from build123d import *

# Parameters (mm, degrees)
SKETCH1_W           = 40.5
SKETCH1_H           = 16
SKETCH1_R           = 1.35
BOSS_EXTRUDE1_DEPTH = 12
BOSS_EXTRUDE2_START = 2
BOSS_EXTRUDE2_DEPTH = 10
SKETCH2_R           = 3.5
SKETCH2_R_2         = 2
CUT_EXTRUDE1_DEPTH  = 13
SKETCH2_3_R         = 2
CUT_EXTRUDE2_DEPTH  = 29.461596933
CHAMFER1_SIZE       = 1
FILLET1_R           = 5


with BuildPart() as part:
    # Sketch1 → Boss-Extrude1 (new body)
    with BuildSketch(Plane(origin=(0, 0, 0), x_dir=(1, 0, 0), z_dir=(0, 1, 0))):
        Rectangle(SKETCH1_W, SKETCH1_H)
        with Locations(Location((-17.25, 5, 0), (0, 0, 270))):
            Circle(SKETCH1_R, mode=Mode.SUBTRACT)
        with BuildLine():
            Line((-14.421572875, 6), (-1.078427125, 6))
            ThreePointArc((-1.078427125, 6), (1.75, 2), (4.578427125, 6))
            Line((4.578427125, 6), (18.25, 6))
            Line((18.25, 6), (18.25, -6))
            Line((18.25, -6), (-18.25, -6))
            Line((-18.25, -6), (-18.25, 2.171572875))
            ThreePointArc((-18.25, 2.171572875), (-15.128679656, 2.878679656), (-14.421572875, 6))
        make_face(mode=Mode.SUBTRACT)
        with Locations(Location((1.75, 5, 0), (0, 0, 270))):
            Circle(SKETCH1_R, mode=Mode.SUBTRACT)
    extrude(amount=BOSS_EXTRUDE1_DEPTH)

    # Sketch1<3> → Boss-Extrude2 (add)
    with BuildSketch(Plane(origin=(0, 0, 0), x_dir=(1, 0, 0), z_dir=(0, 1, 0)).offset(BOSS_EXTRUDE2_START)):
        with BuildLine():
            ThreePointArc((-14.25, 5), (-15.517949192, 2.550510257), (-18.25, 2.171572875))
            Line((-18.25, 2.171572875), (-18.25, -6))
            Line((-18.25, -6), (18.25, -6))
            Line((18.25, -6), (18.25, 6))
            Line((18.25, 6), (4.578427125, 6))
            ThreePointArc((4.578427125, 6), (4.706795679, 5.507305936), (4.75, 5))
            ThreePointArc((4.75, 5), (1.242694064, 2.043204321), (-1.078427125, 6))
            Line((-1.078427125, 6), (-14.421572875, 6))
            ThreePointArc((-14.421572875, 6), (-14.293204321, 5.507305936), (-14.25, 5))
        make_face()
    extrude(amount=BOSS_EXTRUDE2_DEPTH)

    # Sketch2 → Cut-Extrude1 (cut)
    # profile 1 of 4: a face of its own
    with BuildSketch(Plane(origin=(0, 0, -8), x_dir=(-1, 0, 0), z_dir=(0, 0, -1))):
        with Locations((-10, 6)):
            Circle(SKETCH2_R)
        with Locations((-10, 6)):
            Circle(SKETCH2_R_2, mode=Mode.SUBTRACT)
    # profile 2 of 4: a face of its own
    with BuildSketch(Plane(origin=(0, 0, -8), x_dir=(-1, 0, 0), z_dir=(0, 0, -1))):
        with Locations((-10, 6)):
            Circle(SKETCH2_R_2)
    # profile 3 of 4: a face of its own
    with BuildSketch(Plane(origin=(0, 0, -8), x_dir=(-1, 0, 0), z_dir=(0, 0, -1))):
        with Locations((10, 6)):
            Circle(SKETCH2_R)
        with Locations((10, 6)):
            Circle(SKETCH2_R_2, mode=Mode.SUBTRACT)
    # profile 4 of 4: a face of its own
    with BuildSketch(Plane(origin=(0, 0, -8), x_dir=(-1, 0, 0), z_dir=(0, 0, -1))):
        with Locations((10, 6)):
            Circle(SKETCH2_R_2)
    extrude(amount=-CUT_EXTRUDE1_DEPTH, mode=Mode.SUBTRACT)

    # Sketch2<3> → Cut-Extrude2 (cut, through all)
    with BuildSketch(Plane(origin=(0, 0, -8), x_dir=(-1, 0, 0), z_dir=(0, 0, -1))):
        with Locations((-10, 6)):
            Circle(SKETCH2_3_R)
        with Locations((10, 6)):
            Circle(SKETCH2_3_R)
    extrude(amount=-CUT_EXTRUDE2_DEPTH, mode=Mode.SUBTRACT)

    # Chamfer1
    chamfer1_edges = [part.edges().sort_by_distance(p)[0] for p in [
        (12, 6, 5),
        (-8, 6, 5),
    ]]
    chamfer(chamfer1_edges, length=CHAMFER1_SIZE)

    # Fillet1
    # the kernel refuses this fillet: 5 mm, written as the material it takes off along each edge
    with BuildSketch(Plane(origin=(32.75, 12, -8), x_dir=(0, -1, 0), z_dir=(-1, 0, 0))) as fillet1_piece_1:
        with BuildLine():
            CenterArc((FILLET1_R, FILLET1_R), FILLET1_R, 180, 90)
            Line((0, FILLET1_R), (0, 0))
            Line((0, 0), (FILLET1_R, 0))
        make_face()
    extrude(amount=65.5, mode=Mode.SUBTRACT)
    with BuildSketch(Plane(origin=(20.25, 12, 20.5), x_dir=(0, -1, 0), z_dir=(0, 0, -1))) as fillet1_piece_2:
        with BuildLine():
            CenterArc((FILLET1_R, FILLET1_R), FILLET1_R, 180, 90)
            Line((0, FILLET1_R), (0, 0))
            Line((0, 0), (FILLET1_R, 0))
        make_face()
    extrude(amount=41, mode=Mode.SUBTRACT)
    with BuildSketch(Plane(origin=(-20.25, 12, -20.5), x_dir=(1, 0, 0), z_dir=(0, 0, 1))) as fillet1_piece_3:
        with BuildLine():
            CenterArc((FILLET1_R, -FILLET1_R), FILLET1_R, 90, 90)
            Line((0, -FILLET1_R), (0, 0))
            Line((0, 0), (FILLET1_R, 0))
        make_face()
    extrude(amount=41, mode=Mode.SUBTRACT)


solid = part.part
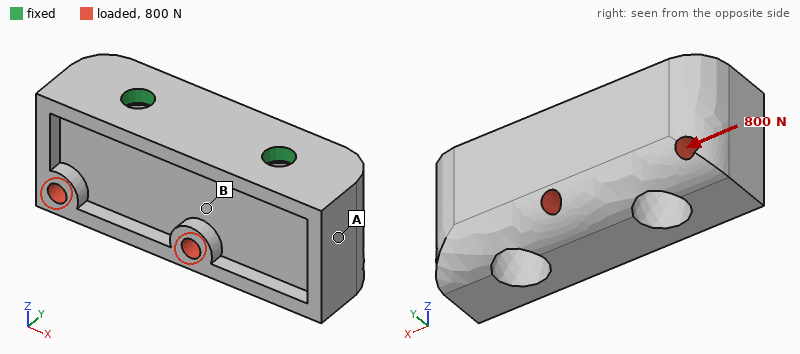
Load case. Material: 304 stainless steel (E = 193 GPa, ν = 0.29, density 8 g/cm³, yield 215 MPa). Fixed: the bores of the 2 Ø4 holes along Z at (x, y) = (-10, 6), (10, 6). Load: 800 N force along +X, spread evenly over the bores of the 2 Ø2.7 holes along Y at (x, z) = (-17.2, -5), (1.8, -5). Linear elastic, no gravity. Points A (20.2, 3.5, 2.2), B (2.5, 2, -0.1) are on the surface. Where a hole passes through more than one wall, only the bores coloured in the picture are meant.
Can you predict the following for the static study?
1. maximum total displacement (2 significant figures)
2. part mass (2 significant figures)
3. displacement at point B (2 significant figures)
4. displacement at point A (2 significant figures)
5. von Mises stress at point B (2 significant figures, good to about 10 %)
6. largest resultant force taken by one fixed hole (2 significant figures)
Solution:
4.0 µm
43 g
1.1 µm
1.6 µm
14 MPa
620 N
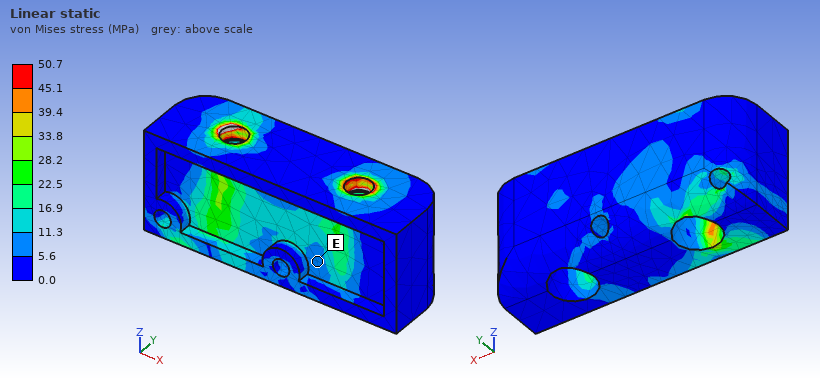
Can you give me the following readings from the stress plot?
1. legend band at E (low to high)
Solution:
5.6 to 11.3 MPa
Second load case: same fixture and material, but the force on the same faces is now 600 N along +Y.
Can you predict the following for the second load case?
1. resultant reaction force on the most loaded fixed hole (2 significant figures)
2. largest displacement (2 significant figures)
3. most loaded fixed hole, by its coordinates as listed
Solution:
480 N
17 µm
(-10, 6)
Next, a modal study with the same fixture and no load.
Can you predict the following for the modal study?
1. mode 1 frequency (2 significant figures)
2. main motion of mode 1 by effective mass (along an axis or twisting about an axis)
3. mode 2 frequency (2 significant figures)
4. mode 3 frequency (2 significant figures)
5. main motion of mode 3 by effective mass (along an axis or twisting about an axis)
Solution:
8100 Hz
along Y
16 kHz
19 kHz
along X
